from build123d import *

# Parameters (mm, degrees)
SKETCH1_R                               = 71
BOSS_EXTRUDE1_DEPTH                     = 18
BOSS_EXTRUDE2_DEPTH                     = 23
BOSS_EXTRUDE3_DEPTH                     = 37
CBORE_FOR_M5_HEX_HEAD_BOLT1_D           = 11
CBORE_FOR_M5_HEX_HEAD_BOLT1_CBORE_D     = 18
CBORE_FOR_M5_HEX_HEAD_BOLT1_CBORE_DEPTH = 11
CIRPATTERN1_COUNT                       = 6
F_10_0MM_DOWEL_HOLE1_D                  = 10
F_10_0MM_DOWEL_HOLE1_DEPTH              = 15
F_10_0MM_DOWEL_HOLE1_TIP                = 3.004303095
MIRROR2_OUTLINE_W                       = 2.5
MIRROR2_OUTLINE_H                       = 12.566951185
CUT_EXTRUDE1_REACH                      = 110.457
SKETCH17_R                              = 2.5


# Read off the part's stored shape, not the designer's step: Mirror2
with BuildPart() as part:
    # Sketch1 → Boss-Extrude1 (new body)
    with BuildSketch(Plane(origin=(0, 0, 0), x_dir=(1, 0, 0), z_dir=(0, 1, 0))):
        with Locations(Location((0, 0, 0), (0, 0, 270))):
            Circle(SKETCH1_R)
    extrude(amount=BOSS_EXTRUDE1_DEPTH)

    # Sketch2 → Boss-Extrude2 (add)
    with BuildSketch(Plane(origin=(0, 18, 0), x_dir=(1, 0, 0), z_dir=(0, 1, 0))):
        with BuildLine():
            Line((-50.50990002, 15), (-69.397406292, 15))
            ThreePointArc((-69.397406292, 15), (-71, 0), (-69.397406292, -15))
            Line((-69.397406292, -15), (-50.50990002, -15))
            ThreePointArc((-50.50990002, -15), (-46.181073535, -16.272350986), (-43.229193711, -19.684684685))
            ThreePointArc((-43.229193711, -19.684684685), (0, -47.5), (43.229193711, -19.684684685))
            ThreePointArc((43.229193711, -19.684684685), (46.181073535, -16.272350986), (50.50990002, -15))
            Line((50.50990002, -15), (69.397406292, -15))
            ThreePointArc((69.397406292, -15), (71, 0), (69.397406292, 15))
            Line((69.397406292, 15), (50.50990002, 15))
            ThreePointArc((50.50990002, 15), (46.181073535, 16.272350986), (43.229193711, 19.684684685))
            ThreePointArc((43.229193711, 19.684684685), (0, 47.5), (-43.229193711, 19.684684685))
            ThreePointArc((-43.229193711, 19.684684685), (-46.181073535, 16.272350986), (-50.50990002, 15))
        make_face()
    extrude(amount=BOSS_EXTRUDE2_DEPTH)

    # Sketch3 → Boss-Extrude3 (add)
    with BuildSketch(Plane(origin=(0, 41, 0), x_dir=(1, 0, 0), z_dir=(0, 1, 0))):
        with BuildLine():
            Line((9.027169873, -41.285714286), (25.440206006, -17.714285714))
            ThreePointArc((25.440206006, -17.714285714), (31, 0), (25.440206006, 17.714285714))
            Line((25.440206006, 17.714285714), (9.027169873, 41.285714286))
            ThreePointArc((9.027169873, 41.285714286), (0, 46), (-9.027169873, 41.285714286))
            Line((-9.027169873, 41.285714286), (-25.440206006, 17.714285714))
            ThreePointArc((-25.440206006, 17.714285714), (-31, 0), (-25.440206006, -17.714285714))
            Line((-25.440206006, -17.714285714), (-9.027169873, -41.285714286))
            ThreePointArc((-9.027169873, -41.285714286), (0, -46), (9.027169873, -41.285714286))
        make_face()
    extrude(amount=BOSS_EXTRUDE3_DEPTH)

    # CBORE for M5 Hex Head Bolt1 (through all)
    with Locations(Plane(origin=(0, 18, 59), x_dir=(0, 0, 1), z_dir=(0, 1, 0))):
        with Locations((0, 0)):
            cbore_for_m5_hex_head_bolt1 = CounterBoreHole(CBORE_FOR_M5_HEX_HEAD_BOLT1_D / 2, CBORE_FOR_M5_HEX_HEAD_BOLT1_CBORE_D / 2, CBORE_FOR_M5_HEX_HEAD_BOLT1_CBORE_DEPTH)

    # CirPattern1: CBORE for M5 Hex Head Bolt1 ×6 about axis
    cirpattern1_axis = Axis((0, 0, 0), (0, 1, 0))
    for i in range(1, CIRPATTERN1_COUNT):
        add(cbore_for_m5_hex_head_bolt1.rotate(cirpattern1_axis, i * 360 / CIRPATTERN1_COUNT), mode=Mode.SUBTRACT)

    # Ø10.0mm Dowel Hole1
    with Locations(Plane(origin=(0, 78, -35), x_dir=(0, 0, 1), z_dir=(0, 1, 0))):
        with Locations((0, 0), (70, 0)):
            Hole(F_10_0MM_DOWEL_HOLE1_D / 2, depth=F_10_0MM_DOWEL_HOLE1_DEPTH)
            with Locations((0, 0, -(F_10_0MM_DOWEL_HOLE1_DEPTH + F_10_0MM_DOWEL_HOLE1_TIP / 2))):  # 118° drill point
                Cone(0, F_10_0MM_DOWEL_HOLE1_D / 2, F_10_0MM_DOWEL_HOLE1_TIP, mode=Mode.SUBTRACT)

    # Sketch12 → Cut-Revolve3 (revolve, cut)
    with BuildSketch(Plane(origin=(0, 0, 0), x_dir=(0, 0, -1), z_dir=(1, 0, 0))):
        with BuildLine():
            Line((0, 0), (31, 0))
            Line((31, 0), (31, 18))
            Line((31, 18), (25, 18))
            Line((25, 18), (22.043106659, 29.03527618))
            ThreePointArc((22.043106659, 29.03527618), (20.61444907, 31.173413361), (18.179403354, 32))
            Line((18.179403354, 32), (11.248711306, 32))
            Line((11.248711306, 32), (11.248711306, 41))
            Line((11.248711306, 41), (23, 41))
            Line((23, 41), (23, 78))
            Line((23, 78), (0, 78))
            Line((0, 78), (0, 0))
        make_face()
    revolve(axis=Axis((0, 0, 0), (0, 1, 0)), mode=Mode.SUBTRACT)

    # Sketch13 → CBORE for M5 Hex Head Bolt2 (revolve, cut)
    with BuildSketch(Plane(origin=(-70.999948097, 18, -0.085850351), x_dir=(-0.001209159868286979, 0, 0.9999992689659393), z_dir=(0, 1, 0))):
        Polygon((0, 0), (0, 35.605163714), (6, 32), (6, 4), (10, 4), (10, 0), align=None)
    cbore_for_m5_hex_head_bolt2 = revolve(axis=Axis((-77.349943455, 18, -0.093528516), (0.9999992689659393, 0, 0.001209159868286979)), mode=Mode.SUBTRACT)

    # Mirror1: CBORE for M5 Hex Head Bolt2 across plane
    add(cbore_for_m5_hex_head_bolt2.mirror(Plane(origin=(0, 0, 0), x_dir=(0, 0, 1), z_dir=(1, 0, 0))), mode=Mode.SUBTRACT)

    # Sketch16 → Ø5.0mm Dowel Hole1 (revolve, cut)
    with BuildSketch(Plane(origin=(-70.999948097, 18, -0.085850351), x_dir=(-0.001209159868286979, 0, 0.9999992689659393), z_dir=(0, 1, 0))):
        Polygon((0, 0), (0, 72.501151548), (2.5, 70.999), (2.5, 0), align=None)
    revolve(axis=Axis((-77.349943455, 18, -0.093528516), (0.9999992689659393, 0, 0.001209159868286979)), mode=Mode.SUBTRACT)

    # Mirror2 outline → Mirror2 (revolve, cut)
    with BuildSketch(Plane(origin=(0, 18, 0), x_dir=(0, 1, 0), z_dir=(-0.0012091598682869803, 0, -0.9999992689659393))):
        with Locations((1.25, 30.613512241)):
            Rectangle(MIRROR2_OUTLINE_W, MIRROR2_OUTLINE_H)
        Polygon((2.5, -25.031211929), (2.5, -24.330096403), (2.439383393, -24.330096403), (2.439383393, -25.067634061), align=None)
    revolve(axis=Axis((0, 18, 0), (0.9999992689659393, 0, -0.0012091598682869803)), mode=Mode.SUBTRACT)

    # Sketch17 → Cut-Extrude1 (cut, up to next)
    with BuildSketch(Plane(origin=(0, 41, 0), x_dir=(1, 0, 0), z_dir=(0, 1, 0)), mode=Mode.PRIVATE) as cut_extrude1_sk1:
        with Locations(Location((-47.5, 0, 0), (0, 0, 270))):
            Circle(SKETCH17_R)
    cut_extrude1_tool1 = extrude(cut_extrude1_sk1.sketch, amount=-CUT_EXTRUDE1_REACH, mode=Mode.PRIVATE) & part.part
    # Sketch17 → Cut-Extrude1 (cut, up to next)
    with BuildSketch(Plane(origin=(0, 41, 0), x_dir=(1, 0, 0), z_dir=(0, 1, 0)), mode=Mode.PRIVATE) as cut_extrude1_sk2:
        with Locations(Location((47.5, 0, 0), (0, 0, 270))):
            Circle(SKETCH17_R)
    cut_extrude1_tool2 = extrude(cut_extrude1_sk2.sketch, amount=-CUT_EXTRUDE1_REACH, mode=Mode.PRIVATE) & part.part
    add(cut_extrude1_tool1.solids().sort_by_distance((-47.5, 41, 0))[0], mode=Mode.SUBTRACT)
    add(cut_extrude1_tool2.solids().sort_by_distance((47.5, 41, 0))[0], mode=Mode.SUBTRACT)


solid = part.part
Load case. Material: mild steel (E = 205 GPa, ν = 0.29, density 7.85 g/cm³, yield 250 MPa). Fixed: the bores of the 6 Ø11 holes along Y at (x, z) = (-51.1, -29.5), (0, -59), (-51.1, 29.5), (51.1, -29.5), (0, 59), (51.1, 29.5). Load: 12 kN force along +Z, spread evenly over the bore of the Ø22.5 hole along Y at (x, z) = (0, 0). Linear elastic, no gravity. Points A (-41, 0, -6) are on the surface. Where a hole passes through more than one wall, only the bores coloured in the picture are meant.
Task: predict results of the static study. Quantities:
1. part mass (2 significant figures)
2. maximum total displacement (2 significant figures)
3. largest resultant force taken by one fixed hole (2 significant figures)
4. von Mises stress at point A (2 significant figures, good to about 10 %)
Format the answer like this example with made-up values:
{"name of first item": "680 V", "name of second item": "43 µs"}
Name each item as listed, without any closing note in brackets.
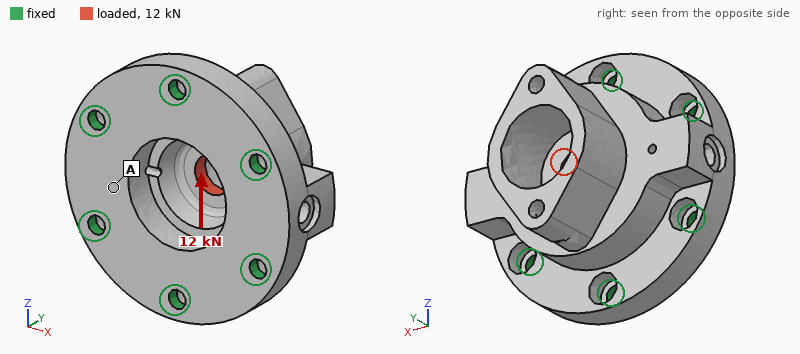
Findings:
{"part mass": "3.5 kg", "maximum total displacement": "4.2 µm", "largest resultant force taken by one fixed hole": "3.4 kN", "von Mises stress at point A": "3.2 MPa"}
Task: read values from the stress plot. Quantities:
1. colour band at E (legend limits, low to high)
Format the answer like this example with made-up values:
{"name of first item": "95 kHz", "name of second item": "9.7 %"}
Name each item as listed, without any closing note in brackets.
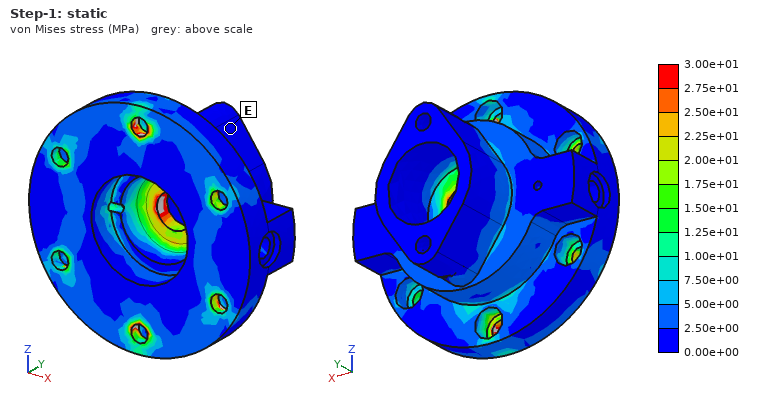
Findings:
{"colour band at E": "0.00e+00 to 2.50e+00 MPa"}
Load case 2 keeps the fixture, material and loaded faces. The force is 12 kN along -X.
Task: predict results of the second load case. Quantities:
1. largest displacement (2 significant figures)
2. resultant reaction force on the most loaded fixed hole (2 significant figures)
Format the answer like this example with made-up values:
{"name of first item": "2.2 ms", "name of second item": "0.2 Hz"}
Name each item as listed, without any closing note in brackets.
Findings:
{"largest displacement": "4.2 µm", "resultant reaction force on the most loaded fixed hole": "3.0 kN"}
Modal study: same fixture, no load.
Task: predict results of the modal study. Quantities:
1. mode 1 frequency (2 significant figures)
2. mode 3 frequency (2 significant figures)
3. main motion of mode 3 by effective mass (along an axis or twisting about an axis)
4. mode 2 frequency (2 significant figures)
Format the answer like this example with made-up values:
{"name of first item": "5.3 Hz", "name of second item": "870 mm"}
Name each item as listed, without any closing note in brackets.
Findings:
{"mode 1 frequency": "6800 Hz", "mode 3 frequency": "8100 Hz", "main motion of mode 3 by effective mass": "along Y", "mode 2 frequency": "6900 Hz"}
